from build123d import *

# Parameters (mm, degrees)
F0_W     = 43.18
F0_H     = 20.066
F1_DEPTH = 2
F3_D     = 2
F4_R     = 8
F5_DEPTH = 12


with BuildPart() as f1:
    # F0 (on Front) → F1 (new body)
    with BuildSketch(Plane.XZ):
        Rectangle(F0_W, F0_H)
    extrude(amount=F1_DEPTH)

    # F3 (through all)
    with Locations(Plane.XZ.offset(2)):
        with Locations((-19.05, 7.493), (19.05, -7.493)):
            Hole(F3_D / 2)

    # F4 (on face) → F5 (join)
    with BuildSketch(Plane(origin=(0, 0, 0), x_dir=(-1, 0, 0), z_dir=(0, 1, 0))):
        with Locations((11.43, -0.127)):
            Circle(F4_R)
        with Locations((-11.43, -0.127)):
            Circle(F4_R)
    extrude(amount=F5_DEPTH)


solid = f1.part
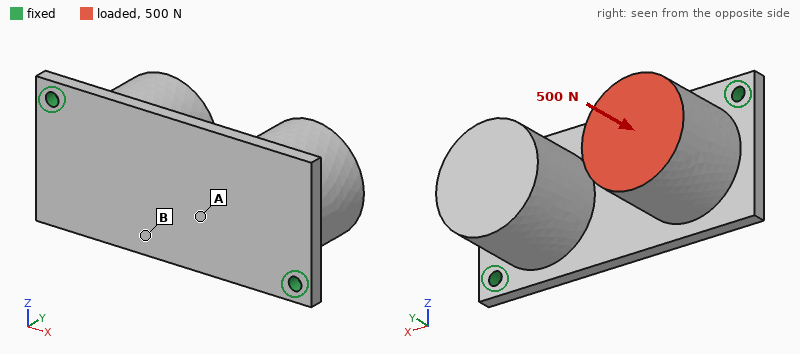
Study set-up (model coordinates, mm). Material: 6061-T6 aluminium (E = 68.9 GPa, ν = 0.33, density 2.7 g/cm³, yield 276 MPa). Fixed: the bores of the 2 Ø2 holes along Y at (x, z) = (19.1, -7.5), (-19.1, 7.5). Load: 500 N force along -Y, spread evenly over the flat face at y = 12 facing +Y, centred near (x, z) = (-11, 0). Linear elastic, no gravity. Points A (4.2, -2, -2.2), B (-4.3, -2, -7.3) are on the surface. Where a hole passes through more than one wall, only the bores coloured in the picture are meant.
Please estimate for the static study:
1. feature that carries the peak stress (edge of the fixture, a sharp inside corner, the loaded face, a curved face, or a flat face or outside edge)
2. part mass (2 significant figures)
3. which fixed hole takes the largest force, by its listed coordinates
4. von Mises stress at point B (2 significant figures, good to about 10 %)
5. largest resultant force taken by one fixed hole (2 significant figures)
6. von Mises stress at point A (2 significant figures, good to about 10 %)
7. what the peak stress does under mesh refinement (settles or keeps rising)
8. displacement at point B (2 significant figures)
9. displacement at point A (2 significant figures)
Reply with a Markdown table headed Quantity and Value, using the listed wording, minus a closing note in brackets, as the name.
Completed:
| Quantity | Value |
|---|---|
| feature that carries the peak stress | edge of the fixture |
| part mass | 18 g |
| which fixed hole takes the largest force, by its listed coordinates | (-19.1, 7.5) |
| von Mises stress at point B | 110 MPa |
| largest resultant force taken by one fixed hole | 390 N |
| von Mises stress at point A | 34 MPa |
| what the peak stress does under mesh refinement | keeps rising |
| displacement at point B | 0.16 mm |
| displacement at point A | 0.086 mm |
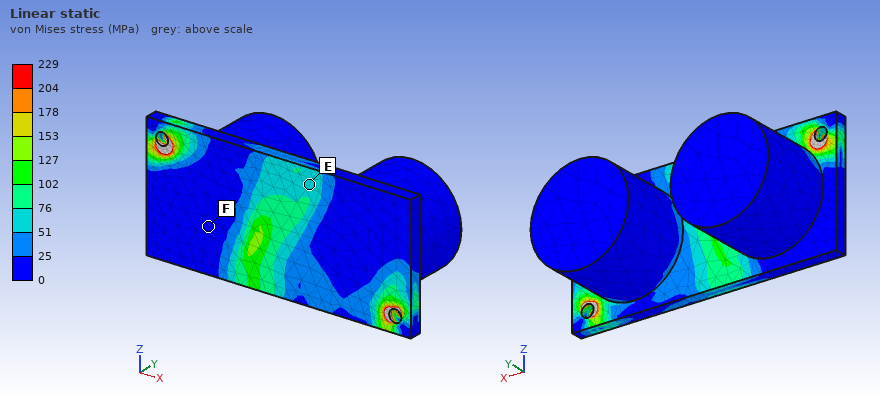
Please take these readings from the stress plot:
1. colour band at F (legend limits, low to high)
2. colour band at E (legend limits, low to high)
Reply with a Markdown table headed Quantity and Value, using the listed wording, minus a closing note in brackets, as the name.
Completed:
| Quantity | Value |
|---|---|
| colour band at F | 0 to 25 MPa |
| colour band at E | 51 to 76 MPa |
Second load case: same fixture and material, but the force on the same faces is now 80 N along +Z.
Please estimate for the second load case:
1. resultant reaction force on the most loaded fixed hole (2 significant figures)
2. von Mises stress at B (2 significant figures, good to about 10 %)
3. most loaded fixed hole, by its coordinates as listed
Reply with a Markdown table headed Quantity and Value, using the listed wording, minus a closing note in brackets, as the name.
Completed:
| Quantity | Value |
|---|---|
| resultant reaction force on the most loaded fixed hole | 66 N |
| von Mises stress at B | 18 MPa |
| most loaded fixed hole, by its coordinates as listed | (-19.1, 7.5) |
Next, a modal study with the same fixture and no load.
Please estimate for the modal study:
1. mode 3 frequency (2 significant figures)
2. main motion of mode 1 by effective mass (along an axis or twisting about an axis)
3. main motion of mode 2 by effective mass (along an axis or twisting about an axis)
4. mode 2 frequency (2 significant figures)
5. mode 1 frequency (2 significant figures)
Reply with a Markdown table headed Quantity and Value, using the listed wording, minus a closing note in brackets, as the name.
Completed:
| Quantity | Value |
|---|---|
| mode 3 frequency | 4800 Hz |
| main motion of mode 1 by effective mass | along Z |
| main motion of mode 2 by effective mass | along Y |
| mode 2 frequency | 2700 Hz |
| mode 1 frequency | 2500 Hz |
